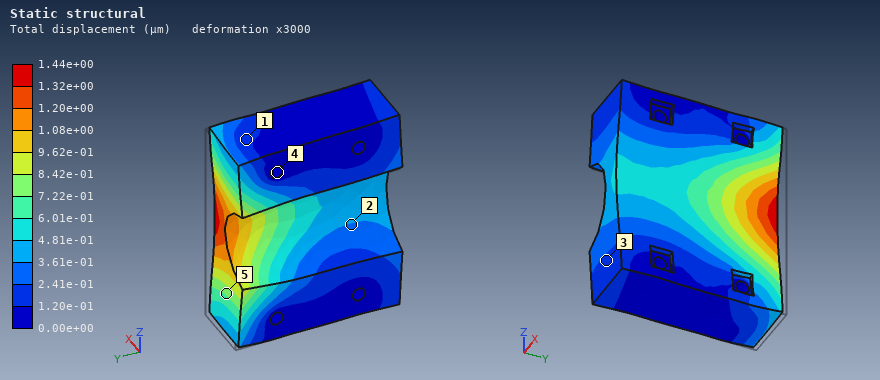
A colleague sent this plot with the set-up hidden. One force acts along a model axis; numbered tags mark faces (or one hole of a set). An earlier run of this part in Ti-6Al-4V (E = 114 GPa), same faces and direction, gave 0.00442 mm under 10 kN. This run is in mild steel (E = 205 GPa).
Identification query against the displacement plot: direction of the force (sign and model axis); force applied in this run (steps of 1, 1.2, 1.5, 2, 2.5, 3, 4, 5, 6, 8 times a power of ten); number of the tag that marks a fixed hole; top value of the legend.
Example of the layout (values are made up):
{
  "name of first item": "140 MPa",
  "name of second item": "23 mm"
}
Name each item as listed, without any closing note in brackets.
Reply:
{
  "direction of the force": "-Y",
  "force applied in this run": "6 kN",
  "number of the tag that marks a fixed hole": "4",
  "top value of the legend": "1.44e+00 µm"
}
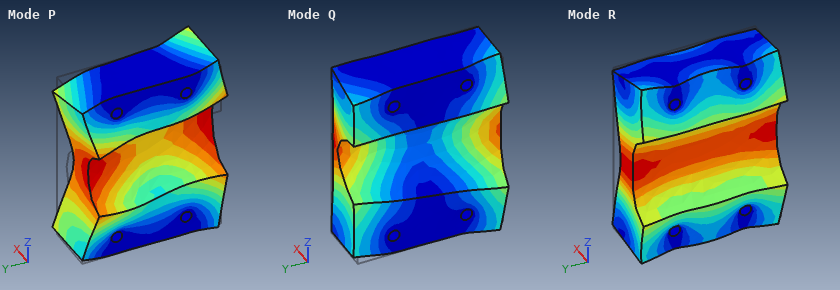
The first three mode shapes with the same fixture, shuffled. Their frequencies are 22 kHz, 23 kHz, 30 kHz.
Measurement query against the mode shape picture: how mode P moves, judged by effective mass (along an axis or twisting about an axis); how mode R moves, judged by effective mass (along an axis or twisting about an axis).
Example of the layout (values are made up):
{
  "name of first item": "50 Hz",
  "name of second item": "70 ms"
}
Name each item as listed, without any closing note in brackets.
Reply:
{
  "how mode P moves, judged by effective mass": "along Y",
  "how mode R moves, judged by effective mass": "along X"
}
